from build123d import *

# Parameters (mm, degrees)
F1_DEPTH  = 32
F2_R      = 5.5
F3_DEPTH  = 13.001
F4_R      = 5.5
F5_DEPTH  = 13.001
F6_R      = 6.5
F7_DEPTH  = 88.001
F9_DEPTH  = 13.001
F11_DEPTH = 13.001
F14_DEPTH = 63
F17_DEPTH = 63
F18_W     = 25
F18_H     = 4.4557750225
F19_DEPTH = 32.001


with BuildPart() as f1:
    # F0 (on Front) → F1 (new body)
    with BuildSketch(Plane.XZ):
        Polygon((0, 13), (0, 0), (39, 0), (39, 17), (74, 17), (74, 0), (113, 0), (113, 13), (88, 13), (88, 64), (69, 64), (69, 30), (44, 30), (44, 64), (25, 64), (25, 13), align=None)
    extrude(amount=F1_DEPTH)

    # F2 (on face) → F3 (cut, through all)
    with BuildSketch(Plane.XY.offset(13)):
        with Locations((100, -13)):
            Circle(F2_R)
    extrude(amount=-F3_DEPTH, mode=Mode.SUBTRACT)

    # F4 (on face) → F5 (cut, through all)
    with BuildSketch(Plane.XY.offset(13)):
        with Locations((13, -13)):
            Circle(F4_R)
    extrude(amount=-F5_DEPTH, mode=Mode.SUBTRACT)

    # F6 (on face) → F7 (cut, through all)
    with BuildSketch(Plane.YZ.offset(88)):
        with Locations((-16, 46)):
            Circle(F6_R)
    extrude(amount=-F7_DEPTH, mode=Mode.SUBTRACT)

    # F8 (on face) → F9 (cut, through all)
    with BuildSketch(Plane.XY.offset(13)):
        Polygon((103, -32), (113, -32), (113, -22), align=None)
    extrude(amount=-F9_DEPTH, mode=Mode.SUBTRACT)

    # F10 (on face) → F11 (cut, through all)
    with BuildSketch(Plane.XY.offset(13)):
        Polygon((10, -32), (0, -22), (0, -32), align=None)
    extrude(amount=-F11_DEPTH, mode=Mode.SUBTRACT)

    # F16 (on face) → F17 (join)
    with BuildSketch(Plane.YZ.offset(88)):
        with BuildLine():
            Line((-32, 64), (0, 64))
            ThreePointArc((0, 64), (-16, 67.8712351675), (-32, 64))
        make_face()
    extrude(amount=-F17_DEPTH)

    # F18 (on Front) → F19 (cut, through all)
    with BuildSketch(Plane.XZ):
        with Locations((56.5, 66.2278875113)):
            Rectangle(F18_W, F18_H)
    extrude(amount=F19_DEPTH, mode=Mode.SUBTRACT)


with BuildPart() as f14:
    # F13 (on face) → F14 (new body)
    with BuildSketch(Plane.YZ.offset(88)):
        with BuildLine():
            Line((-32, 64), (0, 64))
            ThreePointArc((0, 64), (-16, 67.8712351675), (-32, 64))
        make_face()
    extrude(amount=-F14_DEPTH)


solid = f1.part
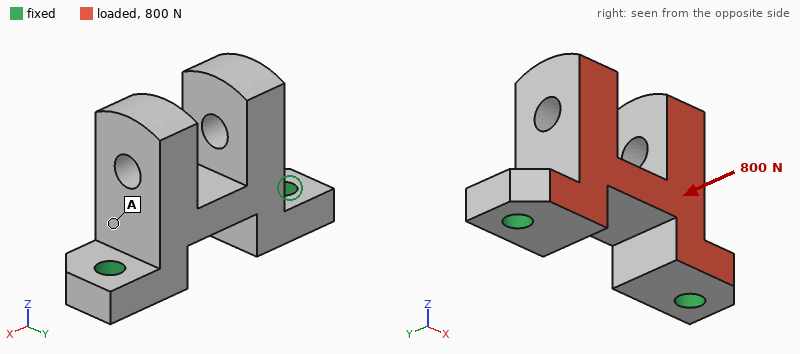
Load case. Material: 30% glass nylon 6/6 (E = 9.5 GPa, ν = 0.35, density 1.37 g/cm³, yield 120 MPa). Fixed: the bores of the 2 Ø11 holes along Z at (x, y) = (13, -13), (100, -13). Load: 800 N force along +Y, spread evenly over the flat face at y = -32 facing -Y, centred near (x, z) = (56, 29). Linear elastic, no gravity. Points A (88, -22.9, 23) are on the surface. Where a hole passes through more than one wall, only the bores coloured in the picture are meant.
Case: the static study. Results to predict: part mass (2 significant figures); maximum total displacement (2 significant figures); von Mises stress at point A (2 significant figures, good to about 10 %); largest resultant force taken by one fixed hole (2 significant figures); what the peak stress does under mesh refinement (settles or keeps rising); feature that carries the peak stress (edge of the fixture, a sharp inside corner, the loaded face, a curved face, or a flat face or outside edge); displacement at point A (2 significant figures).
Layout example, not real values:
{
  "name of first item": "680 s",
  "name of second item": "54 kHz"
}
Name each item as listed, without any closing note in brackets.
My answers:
{
  "part mass": "130 g",
  "maximum total displacement": "0.13 mm",
  "von Mises stress at point A": "2.3 MPa",
  "largest resultant force taken by one fixed hole": "400 N",
  "what the peak stress does under mesh refinement": "keeps rising",
  "feature that carries the peak stress": "edge of the fixture",
  "displacement at point A": "0.042 mm"
}
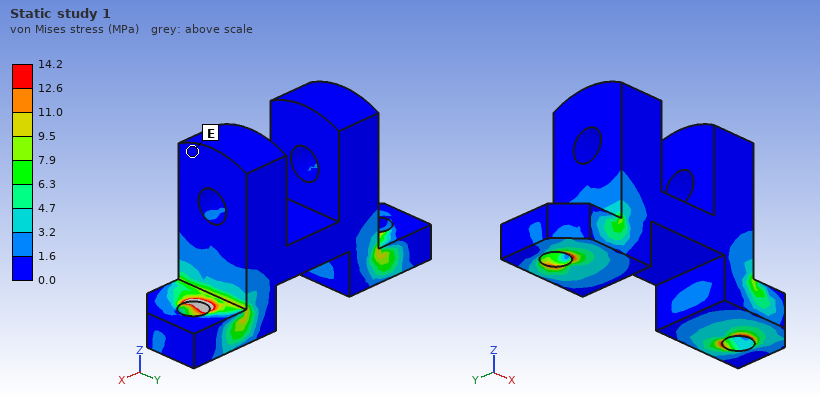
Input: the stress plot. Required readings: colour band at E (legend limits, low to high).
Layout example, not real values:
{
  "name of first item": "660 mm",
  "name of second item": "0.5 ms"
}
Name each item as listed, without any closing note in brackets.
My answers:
{
  "colour band at E": "0.0 to 1.6 MPa"
}
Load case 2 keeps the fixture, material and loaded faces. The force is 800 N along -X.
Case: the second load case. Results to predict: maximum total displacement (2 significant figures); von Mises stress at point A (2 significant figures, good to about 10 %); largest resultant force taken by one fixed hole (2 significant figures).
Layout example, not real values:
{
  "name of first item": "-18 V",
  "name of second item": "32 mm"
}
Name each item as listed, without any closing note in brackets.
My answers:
{
  "maximum total displacement": "47 µm",
  "von Mises stress at point A": "1.4 MPa",
  "largest resultant force taken by one fixed hole": "480 N"
}
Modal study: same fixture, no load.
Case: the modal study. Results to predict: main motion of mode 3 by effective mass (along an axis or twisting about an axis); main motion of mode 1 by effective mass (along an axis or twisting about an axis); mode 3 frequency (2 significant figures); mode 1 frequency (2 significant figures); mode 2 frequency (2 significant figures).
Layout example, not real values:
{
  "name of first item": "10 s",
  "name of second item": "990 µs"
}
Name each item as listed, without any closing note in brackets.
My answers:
{
  "main motion of mode 3 by effective mass": "along X",
  "main motion of mode 1 by effective mass": "along Y",
  "mode 3 frequency": "2600 Hz",
  "mode 1 frequency": "1300 Hz",
  "mode 2 frequency": "2100 Hz"
}
